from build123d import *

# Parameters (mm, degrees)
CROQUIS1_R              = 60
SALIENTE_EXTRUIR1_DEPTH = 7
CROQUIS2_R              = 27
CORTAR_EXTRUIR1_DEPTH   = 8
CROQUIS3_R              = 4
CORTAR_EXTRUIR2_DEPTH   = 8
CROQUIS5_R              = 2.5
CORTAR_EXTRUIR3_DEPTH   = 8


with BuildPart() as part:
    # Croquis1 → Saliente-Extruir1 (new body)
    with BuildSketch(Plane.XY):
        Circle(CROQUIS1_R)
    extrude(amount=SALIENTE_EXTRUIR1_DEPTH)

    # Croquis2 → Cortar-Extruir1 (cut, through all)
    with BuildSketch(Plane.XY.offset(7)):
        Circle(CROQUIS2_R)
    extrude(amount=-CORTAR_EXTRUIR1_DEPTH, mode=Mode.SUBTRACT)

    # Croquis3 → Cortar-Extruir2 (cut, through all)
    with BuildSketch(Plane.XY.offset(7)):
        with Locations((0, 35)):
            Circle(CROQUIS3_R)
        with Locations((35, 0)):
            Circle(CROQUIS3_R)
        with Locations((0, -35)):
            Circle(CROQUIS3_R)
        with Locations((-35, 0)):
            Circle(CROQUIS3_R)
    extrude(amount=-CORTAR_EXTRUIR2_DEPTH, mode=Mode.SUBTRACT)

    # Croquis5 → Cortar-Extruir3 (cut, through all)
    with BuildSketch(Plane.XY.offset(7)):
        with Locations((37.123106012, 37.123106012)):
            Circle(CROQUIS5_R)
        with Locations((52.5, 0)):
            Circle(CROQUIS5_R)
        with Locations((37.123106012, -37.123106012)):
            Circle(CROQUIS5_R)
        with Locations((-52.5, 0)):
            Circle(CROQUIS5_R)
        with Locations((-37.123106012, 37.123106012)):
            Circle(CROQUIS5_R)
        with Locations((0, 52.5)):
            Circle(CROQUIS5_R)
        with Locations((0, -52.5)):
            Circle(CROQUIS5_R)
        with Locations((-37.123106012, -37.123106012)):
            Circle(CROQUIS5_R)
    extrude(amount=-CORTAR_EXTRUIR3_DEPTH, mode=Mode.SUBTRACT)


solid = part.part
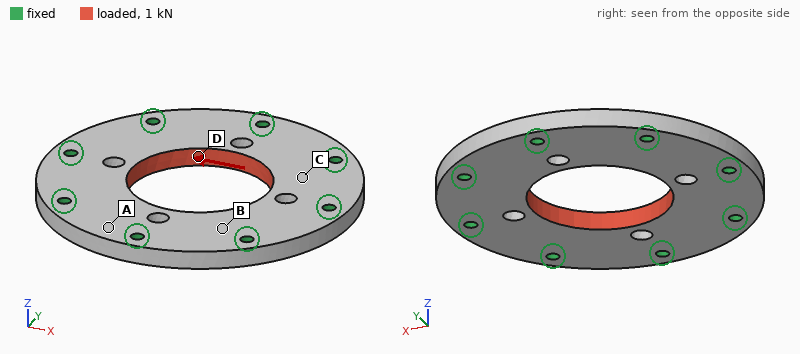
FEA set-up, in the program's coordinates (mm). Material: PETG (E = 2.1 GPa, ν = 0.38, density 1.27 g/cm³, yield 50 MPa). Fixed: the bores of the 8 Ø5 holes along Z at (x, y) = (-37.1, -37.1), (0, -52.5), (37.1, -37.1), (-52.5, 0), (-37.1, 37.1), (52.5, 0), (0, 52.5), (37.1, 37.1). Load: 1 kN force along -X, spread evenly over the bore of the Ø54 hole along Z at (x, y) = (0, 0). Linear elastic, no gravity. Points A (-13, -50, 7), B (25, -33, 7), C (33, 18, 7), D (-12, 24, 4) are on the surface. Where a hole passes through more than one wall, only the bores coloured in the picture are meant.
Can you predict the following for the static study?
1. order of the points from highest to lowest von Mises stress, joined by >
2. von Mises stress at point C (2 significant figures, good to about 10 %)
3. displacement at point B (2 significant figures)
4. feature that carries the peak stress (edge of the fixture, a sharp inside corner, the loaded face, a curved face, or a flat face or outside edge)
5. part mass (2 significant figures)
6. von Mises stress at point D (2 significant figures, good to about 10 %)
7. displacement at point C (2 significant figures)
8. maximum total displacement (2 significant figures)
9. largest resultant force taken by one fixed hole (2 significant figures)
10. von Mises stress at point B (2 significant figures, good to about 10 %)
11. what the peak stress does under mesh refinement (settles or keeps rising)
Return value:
D > B > C > A
0.48 MPa
6.1 µm
edge of the fixture
77 g
1.4 MPa
12 µm
22 µm
180 N
1.0 MPa
keeps rising
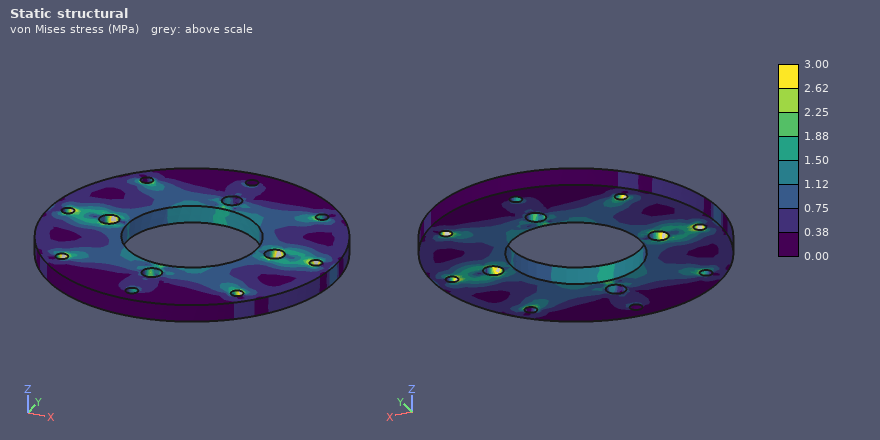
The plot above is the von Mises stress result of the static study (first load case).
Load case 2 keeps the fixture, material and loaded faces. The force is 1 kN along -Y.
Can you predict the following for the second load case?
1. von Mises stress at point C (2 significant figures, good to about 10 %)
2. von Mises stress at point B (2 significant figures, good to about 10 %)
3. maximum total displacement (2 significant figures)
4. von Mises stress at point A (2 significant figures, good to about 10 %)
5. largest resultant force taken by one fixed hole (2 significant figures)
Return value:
0.91 MPa
0.69 MPa
22 µm
0.46 MPa
180 N
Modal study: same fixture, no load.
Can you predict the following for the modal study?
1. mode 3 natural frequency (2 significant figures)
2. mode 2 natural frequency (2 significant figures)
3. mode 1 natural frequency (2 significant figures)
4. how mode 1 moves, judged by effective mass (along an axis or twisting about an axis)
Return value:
2600 Hz
2600 Hz
2200 Hz
along Z
